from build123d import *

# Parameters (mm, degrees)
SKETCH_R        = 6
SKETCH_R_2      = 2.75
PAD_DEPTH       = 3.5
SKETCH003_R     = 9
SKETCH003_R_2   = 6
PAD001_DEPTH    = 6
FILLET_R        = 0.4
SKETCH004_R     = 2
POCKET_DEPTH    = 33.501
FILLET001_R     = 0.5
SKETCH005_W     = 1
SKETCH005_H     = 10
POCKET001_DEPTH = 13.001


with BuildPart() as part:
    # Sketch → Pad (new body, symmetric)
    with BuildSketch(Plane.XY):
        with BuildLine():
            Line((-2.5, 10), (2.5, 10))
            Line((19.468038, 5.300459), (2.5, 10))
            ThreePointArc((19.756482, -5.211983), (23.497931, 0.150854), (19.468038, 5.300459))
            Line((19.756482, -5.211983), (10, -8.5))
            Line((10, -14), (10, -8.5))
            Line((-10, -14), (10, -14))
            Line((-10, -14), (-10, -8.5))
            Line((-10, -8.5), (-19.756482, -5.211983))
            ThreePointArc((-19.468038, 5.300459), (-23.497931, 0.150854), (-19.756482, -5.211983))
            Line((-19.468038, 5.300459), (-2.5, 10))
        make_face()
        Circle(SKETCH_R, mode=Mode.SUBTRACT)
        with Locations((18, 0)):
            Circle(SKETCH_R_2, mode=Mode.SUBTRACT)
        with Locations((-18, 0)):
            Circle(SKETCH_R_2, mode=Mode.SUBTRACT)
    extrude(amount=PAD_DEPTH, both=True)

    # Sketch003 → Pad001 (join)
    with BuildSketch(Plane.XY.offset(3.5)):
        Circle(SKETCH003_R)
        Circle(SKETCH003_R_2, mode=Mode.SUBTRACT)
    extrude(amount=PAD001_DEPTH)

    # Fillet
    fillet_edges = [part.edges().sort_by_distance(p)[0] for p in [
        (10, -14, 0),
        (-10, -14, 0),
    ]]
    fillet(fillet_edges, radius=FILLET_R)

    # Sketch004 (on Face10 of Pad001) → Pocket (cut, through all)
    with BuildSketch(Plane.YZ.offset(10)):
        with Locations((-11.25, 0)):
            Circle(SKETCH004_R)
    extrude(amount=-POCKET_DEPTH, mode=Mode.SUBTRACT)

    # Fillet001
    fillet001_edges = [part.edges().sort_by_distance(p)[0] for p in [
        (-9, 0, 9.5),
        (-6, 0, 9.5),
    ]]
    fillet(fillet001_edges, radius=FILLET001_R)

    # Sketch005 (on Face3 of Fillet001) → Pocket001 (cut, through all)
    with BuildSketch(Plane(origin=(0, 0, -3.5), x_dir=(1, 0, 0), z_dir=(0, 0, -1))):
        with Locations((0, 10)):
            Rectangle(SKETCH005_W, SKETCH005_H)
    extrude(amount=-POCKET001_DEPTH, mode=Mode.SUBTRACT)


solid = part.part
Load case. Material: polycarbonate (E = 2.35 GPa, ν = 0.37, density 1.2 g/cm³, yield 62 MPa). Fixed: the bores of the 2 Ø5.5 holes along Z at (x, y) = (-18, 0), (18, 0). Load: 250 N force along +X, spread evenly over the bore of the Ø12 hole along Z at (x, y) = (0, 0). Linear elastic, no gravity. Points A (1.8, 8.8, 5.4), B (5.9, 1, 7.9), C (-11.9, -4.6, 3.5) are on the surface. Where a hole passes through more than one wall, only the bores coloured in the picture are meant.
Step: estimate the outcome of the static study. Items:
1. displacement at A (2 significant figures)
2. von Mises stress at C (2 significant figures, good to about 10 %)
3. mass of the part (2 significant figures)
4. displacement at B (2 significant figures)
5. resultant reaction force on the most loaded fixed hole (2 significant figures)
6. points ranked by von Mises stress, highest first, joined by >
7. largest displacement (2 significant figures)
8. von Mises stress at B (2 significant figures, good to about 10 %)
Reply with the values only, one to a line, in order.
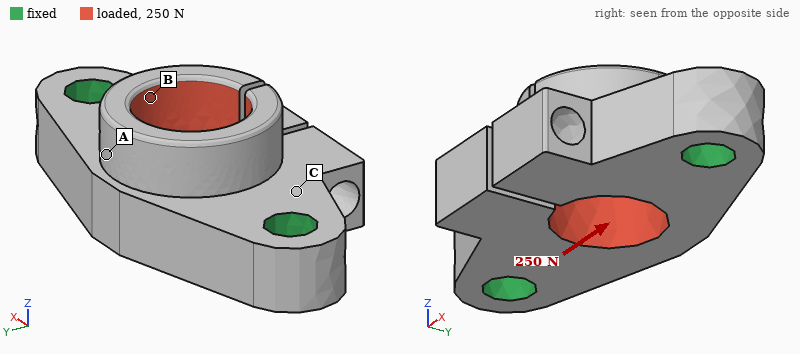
11 µm
2.8 MPa
5.9 g
27 µm
130 N
C > B > A
50 µm
1.7 MPa
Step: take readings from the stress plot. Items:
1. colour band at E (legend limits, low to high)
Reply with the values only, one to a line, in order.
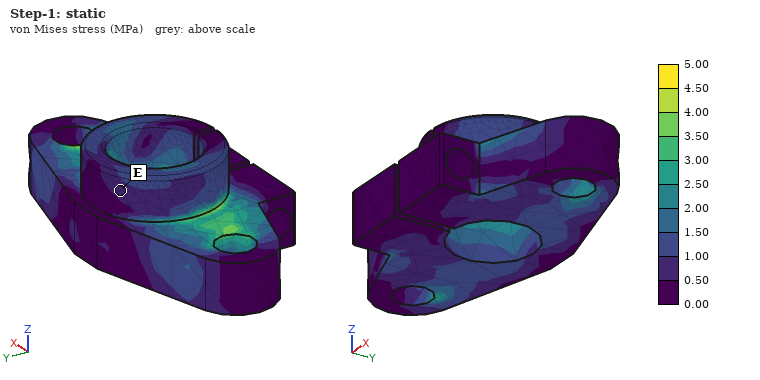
0.50 to 1.00 MPa
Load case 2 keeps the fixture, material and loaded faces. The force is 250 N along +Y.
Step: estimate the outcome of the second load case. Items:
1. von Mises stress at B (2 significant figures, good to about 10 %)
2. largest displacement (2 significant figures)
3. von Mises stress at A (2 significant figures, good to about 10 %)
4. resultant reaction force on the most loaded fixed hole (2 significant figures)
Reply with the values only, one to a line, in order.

1.7 MPa
0.11 mm
1.4 MPa
160 N
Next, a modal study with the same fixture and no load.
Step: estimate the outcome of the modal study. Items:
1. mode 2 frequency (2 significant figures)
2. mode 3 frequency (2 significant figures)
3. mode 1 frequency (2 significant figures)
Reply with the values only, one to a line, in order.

4400 Hz
5100 Hz
4300 Hz
